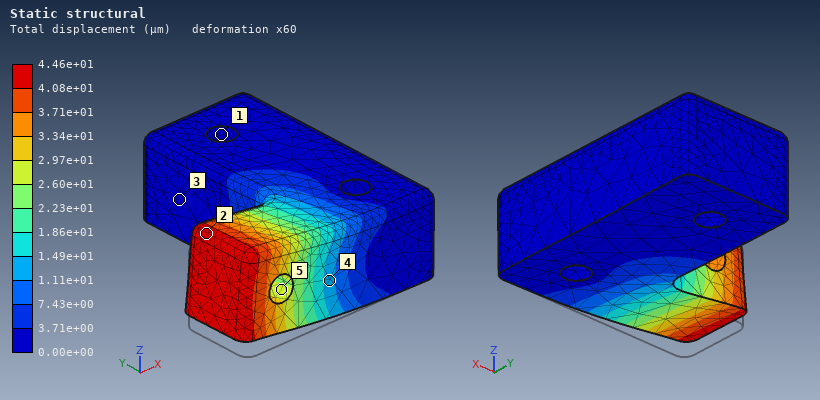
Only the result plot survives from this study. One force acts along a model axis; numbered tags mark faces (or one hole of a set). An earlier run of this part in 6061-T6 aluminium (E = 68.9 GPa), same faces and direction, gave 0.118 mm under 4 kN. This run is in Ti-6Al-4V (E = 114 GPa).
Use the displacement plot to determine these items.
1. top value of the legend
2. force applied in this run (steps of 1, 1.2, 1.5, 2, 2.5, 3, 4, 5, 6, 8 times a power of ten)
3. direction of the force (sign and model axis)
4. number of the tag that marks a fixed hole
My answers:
4.46e+01 µm
2.5 kN
+Z
1
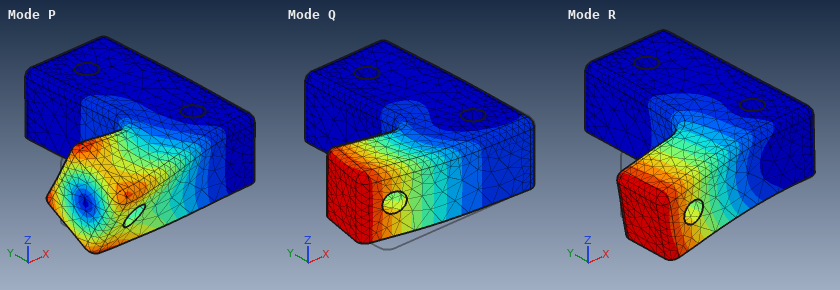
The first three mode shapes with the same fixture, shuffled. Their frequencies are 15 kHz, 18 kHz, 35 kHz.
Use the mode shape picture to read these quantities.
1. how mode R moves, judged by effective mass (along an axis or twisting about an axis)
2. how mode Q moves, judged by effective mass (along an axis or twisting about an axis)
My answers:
along Z
along Y
